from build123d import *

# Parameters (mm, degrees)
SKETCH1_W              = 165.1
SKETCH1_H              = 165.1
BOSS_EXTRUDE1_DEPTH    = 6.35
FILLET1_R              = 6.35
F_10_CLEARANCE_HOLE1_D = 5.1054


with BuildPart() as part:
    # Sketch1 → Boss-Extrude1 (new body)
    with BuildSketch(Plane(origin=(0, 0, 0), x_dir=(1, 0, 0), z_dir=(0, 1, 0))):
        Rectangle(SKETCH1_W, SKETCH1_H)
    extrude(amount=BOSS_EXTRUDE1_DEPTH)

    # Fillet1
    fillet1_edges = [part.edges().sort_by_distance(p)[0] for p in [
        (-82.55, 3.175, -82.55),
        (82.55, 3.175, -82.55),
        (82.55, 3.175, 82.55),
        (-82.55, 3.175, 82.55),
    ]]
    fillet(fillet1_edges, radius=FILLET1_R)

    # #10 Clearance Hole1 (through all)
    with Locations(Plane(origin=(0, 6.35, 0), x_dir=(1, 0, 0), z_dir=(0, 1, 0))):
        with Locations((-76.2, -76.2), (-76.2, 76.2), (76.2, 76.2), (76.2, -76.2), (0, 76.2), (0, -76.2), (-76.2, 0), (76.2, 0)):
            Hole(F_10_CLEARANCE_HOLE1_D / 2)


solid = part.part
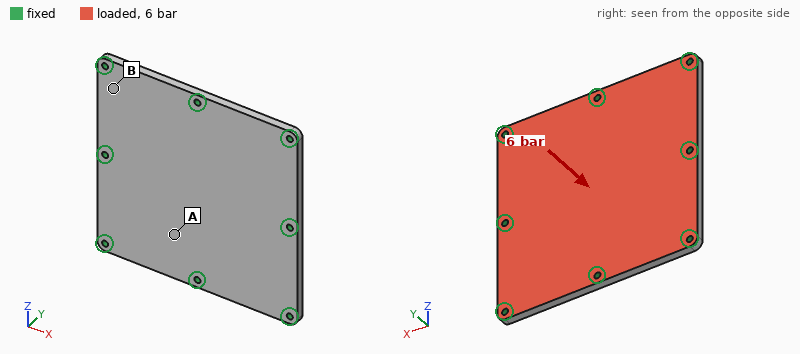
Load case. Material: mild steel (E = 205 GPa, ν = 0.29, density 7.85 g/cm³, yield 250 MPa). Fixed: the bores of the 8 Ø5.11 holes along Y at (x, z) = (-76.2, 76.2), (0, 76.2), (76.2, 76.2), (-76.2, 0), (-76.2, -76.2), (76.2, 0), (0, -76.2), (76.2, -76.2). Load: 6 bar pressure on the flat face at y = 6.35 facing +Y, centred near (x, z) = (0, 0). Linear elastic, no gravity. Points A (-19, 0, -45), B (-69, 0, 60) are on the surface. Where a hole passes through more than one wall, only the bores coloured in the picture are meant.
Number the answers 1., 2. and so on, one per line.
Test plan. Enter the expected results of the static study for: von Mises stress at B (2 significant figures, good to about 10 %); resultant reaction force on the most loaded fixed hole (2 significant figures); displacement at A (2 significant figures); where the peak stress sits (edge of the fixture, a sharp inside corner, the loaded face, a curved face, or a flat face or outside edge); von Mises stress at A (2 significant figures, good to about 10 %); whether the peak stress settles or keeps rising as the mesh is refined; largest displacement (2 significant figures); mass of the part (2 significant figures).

1. 22 MPa
2. 3.1 kN
3. 0.074 mm
4. edge of the fixture
5. 41 MPa
6. keeps rising
7. 0.13 mm
8. 1.3 kg
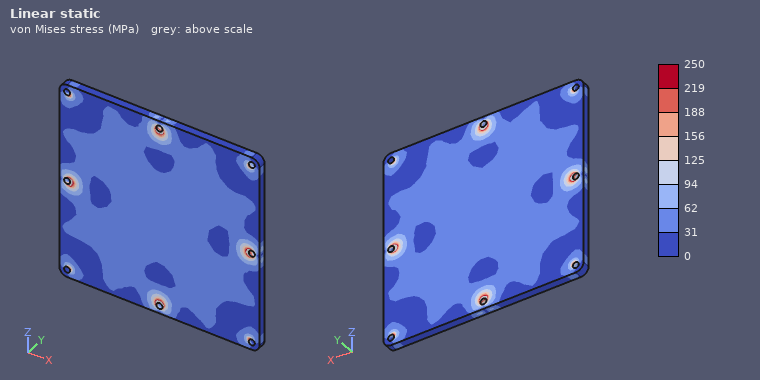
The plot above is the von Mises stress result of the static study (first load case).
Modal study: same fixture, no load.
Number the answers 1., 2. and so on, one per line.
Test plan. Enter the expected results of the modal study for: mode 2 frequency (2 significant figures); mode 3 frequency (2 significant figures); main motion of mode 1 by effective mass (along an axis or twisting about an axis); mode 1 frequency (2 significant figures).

1. 3400 Hz
2. 3400 Hz
3. along Y
4. 1900 Hz
